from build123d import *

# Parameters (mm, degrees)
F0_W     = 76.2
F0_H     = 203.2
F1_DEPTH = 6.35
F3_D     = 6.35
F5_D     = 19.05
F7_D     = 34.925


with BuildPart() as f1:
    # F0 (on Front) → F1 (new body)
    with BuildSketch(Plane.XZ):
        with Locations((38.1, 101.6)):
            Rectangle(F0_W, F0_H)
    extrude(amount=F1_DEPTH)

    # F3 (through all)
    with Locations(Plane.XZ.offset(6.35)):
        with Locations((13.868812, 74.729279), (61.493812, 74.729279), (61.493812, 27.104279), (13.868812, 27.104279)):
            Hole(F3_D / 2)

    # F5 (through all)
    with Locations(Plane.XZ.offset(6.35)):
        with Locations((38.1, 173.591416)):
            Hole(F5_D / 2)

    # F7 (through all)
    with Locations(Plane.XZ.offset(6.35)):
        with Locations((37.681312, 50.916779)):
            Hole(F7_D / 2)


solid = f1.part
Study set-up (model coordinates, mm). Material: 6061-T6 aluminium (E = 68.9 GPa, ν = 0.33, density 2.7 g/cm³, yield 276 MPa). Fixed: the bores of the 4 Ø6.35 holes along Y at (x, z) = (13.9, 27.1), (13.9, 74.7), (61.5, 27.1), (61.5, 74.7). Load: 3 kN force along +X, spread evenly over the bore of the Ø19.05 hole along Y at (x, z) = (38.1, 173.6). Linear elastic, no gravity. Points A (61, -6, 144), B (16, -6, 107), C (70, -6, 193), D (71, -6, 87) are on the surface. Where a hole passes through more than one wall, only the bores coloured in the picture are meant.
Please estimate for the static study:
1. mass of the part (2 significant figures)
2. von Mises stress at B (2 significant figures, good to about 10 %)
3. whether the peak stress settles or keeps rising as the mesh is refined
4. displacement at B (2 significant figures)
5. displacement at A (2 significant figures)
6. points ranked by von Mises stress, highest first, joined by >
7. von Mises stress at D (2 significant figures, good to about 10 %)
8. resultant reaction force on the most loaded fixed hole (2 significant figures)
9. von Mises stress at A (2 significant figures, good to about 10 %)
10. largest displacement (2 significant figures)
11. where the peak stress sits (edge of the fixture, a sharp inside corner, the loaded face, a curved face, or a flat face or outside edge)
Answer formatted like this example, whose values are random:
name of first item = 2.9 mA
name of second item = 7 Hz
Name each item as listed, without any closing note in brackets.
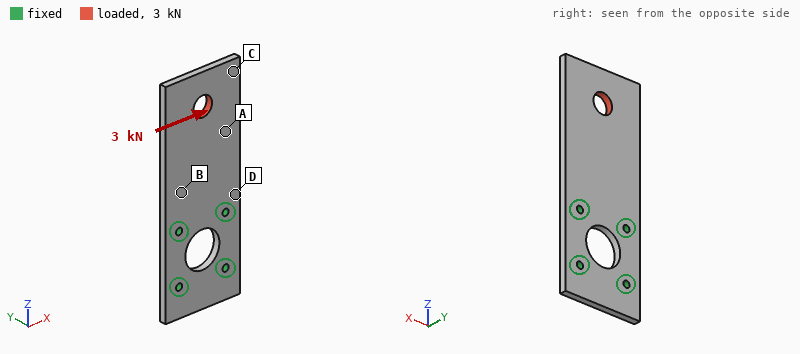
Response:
mass of the part = 240 g
von Mises stress at B = 22 MPa
whether the peak stress settles or keeps rising as the mesh is refined = keeps rising
displacement at B = 0.026 mm
displacement at A = 0.065 mm
points ranked by von Mises stress, highest first, joined by > = D > B > A > C
von Mises stress at D = 32 MPa
resultant reaction force on the most loaded fixed hole = 5.3 kN
von Mises stress at A = 13 MPa
largest displacement = 0.14 mm
where the peak stress sits = edge of the fixture
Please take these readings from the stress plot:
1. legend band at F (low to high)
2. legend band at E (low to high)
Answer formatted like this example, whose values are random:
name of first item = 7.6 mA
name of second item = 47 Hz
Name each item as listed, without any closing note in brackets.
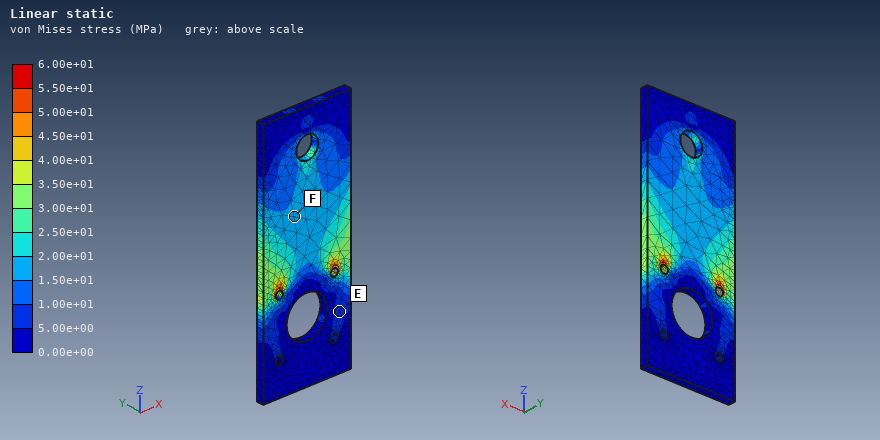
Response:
legend band at F = 1.50e+01 to 2.00e+01 MPa
legend band at E = 5.00e+00 to 1.00e+01 MPa
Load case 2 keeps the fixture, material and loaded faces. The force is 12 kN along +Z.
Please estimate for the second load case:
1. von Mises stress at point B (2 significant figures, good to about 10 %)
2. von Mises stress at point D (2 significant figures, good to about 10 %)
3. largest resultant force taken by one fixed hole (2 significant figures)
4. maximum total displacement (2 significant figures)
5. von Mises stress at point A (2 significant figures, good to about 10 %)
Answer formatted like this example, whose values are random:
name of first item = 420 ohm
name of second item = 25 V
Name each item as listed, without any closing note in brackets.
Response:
von Mises stress at point B = 26 MPa
von Mises stress at point D = 25 MPa
largest resultant force taken by one fixed hole = 5.6 kN
maximum total displacement = 56 µm
von Mises stress at point A = 26 MPa
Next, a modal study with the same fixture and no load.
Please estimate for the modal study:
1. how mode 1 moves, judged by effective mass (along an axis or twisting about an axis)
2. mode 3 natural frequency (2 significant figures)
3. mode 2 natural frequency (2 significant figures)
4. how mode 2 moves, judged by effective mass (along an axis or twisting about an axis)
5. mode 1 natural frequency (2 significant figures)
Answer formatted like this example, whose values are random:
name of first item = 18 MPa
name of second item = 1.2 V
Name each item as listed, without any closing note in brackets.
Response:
how mode 1 moves, judged by effective mass = along Y
mode 3 natural frequency = 1900 Hz
mode 2 natural frequency = 1100 Hz
how mode 2 moves, judged by effective mass = twisting about Z
mode 1 natural frequency = 320 Hz
